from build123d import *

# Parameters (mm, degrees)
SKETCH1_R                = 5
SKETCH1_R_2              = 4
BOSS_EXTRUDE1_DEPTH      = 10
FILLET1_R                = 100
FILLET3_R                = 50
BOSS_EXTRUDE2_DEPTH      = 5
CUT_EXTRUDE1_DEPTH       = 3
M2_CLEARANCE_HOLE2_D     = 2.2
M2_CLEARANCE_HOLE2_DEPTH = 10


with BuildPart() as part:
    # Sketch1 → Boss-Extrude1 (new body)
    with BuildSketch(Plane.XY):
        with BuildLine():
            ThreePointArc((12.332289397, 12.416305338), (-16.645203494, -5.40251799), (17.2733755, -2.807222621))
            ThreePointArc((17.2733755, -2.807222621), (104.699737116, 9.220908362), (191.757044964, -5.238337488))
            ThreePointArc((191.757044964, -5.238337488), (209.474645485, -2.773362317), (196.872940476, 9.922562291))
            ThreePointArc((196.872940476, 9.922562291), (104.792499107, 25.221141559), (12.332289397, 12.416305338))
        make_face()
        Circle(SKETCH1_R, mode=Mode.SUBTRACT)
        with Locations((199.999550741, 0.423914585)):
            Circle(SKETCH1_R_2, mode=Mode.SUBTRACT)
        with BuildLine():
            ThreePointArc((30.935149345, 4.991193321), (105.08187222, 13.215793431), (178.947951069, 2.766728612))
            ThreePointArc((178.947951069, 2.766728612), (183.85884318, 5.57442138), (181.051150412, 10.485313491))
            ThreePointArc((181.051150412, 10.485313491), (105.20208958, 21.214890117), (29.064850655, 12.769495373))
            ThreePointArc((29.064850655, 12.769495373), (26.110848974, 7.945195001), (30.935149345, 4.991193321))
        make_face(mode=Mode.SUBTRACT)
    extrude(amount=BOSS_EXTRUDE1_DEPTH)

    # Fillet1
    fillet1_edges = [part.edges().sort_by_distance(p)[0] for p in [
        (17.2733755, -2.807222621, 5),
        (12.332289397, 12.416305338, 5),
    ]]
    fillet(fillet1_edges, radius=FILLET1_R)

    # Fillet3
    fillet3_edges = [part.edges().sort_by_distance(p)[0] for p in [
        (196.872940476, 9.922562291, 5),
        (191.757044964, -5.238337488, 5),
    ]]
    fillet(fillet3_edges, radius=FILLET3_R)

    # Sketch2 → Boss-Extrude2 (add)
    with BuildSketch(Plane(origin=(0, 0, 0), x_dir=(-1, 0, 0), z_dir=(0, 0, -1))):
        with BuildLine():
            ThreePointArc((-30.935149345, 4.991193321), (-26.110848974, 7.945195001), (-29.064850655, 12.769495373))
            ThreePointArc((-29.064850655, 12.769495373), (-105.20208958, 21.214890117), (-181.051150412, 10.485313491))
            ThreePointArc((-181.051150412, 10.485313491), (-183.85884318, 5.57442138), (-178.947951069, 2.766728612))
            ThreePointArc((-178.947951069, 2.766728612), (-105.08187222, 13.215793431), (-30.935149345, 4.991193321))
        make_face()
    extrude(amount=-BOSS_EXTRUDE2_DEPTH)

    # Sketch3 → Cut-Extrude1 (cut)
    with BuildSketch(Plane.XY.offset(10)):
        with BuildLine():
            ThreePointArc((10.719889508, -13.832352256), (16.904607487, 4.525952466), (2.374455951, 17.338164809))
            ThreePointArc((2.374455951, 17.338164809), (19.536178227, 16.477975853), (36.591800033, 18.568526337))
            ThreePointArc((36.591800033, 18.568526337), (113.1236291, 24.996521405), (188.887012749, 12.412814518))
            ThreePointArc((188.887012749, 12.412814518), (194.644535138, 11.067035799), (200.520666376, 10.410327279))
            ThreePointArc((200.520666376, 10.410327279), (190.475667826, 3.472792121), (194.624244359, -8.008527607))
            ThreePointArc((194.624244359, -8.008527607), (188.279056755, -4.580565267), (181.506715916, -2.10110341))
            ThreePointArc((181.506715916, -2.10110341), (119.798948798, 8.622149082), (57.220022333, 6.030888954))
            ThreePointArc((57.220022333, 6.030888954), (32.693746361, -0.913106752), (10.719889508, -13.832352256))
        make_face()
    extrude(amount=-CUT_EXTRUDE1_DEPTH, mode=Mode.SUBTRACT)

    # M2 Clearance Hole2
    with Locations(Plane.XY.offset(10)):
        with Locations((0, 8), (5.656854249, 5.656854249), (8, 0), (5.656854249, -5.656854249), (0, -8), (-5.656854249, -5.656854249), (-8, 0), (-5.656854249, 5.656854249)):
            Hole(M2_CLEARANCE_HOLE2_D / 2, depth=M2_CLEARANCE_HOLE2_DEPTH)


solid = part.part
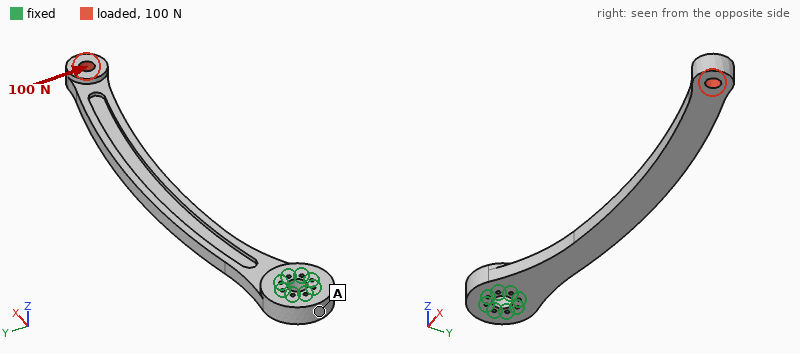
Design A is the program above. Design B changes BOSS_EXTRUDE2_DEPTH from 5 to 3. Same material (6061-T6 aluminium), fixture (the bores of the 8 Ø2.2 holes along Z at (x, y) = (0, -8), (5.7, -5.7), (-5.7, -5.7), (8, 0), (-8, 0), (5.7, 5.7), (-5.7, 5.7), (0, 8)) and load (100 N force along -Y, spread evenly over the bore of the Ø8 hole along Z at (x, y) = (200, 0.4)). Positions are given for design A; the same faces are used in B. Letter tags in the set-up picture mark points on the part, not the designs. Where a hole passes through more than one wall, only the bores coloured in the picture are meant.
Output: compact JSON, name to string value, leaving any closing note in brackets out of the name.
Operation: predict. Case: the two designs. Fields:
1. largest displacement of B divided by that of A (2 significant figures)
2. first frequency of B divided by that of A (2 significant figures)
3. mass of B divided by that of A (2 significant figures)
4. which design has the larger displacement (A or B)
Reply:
{"largest displacement of B divided by that of A": "1.1", "first frequency of B divided by that of A": "1.00", "mass of B divided by that of A": "0.91", "which design has the larger displacement": "B"}
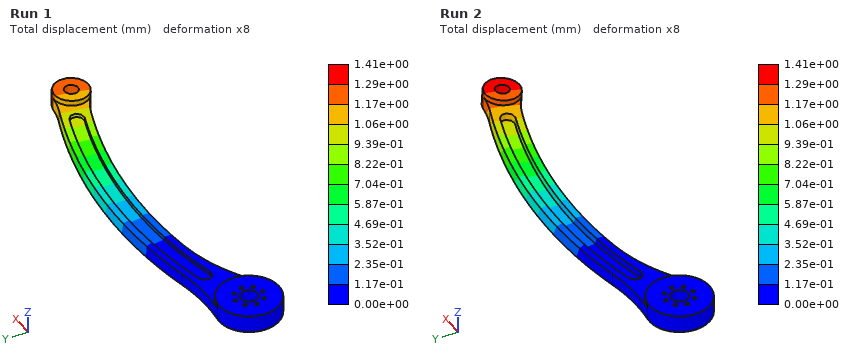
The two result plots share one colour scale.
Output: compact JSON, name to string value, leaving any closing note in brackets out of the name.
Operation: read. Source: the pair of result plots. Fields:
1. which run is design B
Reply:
{"which run is design B": "Run 2"}
